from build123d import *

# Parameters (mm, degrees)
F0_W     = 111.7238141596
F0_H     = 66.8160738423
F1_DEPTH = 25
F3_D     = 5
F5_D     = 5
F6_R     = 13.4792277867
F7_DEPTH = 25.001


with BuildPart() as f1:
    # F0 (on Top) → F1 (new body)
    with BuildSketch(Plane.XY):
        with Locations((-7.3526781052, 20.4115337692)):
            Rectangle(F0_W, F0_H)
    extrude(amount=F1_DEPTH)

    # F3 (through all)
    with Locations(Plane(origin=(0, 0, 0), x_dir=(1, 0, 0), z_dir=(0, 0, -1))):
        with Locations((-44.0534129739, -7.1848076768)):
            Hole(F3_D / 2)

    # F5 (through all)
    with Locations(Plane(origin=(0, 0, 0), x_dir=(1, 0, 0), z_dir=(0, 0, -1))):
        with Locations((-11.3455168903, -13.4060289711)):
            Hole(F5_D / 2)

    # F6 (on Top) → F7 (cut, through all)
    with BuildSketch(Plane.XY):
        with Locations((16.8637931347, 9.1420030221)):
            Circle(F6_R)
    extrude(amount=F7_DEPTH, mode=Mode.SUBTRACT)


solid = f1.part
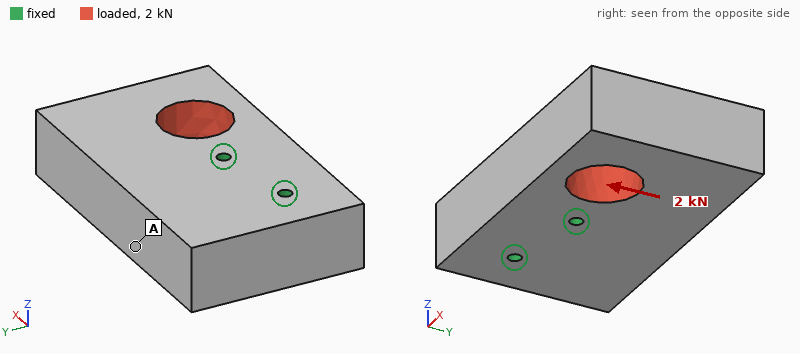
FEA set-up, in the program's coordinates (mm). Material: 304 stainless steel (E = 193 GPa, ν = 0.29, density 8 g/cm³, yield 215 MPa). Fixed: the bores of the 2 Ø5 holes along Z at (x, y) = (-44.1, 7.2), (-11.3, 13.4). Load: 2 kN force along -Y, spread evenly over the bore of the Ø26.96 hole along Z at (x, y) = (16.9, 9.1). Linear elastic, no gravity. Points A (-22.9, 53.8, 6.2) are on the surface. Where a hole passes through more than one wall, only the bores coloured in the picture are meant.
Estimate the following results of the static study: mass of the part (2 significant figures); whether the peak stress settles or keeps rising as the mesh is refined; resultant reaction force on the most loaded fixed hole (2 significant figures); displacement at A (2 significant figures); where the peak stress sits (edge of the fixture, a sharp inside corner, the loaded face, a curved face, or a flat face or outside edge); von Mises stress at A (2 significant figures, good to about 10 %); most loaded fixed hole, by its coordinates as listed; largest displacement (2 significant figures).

1.4 kg
keeps rising
3.5 kN
1.1 µm
edge of the fixture
2.6 MPa
(-11.3, 13.4)
4.0 µm
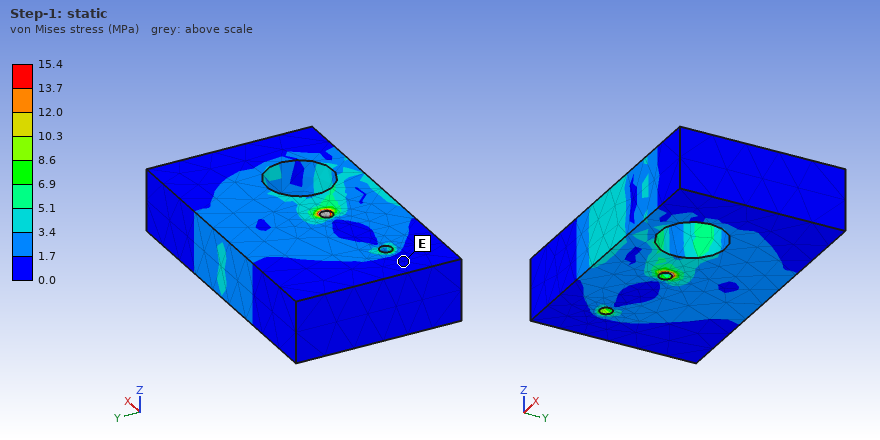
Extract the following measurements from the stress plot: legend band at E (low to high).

0.0 to 1.7 MPa
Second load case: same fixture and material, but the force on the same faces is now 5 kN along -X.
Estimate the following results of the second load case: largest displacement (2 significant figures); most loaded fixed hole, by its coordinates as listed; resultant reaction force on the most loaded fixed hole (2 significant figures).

2.3 µm
(-11.3, 13.4)
3.3 kN
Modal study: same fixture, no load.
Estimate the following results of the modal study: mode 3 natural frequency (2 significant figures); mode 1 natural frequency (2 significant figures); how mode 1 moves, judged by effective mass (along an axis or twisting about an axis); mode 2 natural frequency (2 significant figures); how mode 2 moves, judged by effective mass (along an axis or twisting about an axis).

5300 Hz
3400 Hz
along Z
4600 Hz
along Y
